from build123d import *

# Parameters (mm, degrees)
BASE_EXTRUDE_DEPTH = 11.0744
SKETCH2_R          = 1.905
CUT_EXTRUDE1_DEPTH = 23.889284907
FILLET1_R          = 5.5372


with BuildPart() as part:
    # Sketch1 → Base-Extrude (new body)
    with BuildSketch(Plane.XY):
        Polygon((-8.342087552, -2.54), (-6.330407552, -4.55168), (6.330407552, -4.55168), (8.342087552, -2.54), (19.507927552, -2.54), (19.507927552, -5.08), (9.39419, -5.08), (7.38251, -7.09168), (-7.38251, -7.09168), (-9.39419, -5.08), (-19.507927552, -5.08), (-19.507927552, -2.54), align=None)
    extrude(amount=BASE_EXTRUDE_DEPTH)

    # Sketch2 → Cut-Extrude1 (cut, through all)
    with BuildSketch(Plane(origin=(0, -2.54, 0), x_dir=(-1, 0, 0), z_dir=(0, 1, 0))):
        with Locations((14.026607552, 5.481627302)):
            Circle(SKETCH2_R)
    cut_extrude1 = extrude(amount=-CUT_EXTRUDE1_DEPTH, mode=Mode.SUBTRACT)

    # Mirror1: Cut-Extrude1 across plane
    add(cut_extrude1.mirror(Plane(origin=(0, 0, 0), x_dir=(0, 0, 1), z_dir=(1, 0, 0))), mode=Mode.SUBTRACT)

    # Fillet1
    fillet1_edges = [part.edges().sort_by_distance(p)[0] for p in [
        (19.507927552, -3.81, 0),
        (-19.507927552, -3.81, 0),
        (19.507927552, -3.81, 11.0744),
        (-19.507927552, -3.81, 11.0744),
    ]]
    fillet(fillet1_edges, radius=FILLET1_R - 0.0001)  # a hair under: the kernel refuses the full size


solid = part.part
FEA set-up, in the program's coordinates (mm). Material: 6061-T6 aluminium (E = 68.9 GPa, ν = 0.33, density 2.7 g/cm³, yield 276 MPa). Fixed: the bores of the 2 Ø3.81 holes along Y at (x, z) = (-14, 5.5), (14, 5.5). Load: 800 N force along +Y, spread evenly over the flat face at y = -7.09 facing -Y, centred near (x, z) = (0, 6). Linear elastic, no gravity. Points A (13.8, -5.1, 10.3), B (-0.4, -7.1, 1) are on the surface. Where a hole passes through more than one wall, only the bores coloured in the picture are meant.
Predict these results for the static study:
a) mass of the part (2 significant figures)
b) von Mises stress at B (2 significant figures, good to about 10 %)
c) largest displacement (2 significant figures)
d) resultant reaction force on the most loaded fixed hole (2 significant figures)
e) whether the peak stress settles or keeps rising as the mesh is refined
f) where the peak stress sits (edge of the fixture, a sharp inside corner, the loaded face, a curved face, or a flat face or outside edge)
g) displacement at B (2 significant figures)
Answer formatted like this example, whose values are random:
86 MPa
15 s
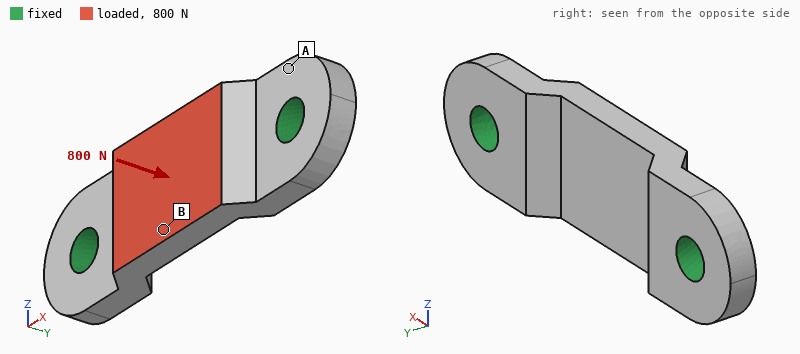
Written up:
2.8 g
94 MPa
34 µm
820 N
keeps rising
edge of the fixture
32 µm
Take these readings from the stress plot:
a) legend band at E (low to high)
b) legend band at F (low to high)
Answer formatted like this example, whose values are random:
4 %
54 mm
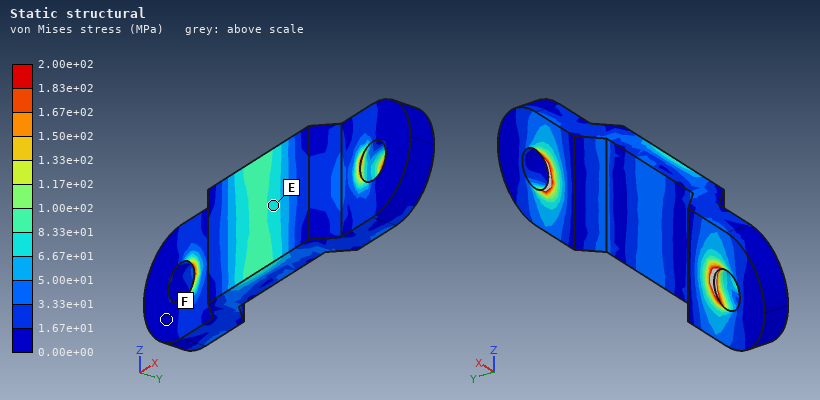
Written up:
6.67e+01 to 8.33e+01 MPa
0.00e+00 to 1.67e+01 MPa
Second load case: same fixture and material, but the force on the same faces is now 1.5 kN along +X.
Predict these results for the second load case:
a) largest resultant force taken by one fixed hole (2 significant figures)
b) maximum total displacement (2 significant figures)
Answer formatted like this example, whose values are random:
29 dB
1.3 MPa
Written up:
780 N
6.9 µm
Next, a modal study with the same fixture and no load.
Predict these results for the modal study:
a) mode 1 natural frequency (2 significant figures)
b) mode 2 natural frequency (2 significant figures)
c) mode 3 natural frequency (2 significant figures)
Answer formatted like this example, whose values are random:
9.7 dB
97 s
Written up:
24 kHz
25 kHz
42 kHz
